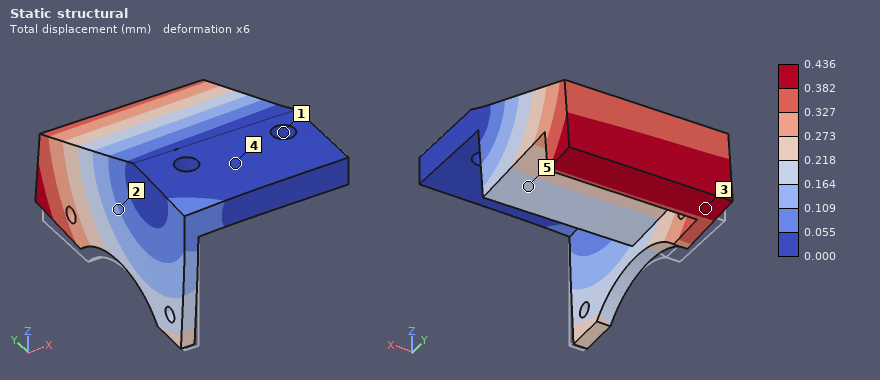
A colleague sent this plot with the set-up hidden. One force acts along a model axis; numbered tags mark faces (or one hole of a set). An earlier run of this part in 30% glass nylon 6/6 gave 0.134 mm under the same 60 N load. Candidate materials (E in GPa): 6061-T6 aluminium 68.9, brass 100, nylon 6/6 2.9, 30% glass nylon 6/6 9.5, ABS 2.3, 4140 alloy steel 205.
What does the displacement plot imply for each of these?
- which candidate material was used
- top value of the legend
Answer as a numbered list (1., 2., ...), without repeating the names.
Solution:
1. nylon 6/6
2. 0.436 mm
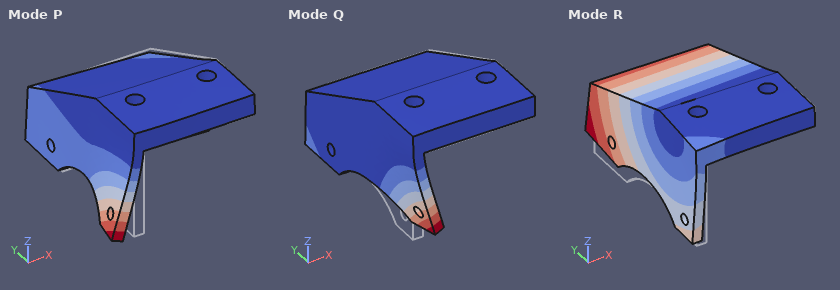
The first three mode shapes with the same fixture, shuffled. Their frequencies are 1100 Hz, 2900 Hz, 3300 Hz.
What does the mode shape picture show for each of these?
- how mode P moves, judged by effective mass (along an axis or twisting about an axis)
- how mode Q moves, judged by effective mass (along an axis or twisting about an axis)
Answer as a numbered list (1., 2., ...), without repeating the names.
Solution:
1. along X
2. along X
